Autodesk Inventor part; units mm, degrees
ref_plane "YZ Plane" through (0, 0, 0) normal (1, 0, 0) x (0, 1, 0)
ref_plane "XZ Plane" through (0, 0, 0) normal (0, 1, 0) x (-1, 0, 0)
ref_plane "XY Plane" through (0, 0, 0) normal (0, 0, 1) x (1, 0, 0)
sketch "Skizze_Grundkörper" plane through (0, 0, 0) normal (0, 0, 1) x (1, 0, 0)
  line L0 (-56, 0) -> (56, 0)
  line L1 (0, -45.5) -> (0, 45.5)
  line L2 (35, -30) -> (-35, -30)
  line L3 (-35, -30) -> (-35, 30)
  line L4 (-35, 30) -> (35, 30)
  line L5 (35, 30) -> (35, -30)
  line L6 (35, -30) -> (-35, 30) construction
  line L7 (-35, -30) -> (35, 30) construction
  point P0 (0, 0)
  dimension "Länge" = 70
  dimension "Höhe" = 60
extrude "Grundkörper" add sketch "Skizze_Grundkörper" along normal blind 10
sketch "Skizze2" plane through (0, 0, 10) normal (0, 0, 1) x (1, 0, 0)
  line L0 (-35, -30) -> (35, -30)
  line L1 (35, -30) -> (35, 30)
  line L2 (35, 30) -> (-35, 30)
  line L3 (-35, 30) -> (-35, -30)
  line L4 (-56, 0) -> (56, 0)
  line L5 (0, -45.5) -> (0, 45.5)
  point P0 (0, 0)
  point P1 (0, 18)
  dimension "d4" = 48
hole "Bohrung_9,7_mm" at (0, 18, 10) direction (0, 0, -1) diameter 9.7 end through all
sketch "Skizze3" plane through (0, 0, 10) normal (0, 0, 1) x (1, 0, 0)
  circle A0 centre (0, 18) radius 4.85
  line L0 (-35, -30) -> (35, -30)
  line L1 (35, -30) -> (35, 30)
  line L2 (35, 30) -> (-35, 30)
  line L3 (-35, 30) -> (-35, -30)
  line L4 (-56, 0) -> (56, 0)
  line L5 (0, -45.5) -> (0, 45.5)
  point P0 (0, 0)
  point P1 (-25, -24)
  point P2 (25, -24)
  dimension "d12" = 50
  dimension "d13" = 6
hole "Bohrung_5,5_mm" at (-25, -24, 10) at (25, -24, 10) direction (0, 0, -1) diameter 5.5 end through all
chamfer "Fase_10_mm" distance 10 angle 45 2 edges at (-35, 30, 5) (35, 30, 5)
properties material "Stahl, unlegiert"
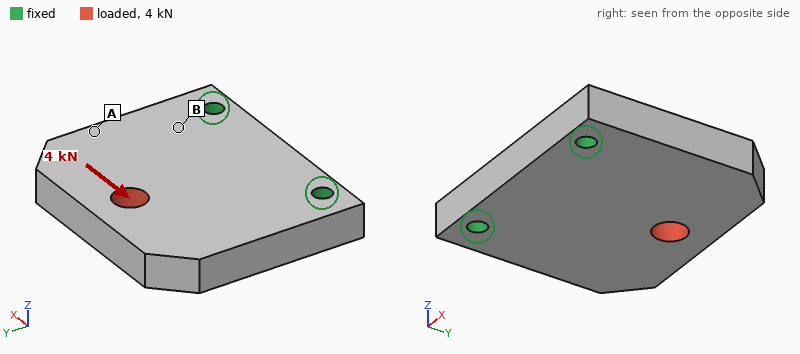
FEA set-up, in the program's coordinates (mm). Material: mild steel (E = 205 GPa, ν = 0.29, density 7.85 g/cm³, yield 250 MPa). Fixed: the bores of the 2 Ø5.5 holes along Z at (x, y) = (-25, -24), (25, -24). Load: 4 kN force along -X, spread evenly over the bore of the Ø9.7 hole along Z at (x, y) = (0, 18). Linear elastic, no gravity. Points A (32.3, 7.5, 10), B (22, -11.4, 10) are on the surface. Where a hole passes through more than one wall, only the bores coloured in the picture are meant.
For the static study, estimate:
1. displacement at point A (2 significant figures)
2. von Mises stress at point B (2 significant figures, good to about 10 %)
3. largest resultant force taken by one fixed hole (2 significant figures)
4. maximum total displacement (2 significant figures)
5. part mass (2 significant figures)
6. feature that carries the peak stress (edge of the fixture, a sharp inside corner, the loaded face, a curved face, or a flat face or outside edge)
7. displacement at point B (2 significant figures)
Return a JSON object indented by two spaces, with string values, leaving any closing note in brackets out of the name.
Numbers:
{
  "displacement at point A": "5.1 µm",
  "von Mises stress at point B": "16 MPa",
  "largest resultant force taken by one fixed hole": "3.7 kN",
  "maximum total displacement": "7.5 µm",
  "part mass": "310 g",
  "feature that carries the peak stress": "edge of the fixture",
  "displacement at point B": "1.8 µm"
}
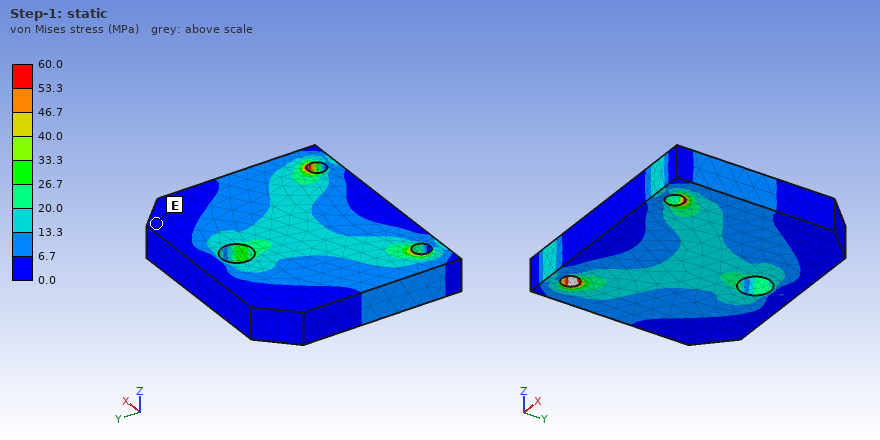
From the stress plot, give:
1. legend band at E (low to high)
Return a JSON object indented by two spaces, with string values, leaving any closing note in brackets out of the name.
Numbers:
{
  "legend band at E": "0.0 to 6.7 MPa"
}
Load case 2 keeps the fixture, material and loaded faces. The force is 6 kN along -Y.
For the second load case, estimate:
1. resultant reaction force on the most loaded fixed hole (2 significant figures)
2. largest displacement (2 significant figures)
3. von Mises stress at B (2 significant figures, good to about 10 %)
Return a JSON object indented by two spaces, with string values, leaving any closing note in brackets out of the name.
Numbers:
{
  "resultant reaction force on the most loaded fixed hole": "3.1 kN",
  "largest displacement": "5.2 µm",
  "von Mises stress at B": "16 MPa"
}
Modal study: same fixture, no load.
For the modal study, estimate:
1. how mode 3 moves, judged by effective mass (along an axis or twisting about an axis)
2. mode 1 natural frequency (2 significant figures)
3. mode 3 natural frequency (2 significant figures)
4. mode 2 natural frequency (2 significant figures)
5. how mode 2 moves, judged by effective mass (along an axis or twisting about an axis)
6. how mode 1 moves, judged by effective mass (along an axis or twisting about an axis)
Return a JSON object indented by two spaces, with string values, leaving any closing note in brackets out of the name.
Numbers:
{
  "how mode 3 moves, judged by effective mass": "along X",
  "mode 1 natural frequency": "2500 Hz",
  "mode 3 natural frequency": "10 kHz",
  "mode 2 natural frequency": "5700 Hz",
  "how mode 2 moves, judged by effective mass": "twisting about Y",
  "how mode 1 moves, judged by effective mass": "along Z"
}
